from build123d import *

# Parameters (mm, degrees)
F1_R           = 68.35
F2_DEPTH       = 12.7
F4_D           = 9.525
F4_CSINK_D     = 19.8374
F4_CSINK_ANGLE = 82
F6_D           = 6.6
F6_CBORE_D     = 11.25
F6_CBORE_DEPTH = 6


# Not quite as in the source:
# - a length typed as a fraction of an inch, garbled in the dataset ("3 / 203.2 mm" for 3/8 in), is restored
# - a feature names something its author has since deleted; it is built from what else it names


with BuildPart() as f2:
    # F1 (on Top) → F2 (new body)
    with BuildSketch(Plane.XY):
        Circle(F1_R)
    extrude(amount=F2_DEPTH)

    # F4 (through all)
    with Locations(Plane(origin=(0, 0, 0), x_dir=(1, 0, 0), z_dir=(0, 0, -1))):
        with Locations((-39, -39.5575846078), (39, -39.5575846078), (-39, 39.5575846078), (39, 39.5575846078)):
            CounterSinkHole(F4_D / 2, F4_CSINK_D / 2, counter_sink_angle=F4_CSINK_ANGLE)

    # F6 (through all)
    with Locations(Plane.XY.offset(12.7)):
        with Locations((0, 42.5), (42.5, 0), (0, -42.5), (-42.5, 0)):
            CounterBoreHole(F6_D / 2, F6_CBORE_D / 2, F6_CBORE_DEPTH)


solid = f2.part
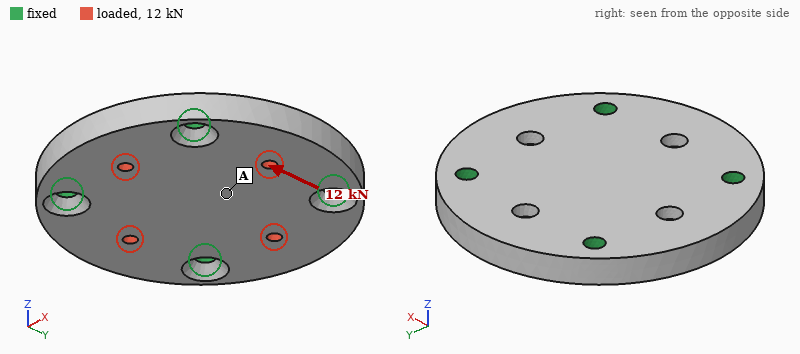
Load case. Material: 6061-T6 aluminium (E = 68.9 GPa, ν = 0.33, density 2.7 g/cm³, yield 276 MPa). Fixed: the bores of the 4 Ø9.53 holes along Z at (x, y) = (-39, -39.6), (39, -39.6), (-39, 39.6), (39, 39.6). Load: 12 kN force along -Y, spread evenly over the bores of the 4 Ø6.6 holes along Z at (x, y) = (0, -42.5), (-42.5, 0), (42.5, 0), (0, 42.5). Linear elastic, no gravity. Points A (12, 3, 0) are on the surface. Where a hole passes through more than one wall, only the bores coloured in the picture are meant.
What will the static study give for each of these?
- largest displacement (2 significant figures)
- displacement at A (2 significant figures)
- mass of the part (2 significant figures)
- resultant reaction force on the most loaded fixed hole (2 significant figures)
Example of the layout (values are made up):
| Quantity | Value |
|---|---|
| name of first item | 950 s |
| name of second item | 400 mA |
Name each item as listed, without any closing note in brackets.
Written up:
| Quantity | Value |
|---|---|
| largest displacement | 10 µm |
| displacement at A | 3.5 µm |
| mass of the part | 480 g |
| resultant reaction force on the most loaded fixed hole | 3.0 kN |
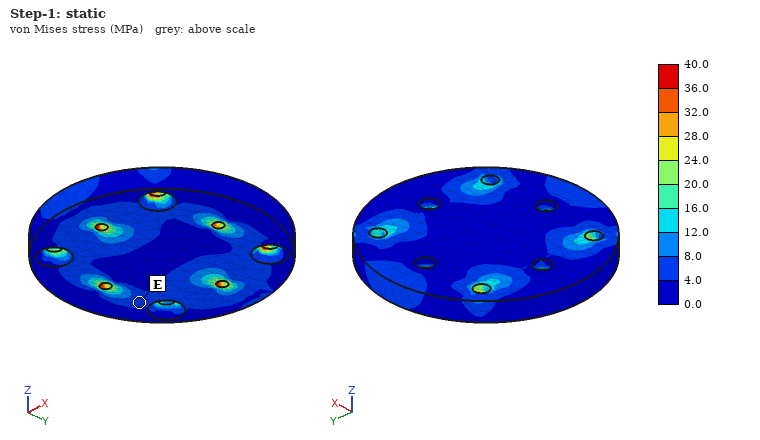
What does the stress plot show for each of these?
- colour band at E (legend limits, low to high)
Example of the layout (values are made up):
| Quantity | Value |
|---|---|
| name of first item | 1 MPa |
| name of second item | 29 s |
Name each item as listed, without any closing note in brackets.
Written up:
| Quantity | Value |
|---|---|
| colour band at E | 4.0 to 8.0 MPa |
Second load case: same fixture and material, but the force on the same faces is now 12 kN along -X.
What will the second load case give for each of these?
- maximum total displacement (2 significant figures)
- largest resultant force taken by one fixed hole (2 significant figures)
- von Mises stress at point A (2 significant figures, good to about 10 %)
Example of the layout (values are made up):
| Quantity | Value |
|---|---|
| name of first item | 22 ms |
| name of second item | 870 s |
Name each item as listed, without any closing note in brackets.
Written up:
| Quantity | Value |
|---|---|
| maximum total displacement | 10 µm |
| largest resultant force taken by one fixed hole | 3.0 kN |
| von Mises stress at point A | 3.6 MPa |
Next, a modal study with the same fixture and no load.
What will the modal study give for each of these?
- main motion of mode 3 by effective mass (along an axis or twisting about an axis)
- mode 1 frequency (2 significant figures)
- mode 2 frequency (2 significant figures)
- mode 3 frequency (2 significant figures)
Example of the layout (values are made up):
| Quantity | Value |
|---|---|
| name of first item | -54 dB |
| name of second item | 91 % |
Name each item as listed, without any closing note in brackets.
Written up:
| Quantity | Value |
|---|---|
| main motion of mode 3 by effective mass | twisting about Y |
| mode 1 frequency | 5900 Hz |
| mode 2 frequency | 6100 Hz |
| mode 3 frequency | 6400 Hz |
